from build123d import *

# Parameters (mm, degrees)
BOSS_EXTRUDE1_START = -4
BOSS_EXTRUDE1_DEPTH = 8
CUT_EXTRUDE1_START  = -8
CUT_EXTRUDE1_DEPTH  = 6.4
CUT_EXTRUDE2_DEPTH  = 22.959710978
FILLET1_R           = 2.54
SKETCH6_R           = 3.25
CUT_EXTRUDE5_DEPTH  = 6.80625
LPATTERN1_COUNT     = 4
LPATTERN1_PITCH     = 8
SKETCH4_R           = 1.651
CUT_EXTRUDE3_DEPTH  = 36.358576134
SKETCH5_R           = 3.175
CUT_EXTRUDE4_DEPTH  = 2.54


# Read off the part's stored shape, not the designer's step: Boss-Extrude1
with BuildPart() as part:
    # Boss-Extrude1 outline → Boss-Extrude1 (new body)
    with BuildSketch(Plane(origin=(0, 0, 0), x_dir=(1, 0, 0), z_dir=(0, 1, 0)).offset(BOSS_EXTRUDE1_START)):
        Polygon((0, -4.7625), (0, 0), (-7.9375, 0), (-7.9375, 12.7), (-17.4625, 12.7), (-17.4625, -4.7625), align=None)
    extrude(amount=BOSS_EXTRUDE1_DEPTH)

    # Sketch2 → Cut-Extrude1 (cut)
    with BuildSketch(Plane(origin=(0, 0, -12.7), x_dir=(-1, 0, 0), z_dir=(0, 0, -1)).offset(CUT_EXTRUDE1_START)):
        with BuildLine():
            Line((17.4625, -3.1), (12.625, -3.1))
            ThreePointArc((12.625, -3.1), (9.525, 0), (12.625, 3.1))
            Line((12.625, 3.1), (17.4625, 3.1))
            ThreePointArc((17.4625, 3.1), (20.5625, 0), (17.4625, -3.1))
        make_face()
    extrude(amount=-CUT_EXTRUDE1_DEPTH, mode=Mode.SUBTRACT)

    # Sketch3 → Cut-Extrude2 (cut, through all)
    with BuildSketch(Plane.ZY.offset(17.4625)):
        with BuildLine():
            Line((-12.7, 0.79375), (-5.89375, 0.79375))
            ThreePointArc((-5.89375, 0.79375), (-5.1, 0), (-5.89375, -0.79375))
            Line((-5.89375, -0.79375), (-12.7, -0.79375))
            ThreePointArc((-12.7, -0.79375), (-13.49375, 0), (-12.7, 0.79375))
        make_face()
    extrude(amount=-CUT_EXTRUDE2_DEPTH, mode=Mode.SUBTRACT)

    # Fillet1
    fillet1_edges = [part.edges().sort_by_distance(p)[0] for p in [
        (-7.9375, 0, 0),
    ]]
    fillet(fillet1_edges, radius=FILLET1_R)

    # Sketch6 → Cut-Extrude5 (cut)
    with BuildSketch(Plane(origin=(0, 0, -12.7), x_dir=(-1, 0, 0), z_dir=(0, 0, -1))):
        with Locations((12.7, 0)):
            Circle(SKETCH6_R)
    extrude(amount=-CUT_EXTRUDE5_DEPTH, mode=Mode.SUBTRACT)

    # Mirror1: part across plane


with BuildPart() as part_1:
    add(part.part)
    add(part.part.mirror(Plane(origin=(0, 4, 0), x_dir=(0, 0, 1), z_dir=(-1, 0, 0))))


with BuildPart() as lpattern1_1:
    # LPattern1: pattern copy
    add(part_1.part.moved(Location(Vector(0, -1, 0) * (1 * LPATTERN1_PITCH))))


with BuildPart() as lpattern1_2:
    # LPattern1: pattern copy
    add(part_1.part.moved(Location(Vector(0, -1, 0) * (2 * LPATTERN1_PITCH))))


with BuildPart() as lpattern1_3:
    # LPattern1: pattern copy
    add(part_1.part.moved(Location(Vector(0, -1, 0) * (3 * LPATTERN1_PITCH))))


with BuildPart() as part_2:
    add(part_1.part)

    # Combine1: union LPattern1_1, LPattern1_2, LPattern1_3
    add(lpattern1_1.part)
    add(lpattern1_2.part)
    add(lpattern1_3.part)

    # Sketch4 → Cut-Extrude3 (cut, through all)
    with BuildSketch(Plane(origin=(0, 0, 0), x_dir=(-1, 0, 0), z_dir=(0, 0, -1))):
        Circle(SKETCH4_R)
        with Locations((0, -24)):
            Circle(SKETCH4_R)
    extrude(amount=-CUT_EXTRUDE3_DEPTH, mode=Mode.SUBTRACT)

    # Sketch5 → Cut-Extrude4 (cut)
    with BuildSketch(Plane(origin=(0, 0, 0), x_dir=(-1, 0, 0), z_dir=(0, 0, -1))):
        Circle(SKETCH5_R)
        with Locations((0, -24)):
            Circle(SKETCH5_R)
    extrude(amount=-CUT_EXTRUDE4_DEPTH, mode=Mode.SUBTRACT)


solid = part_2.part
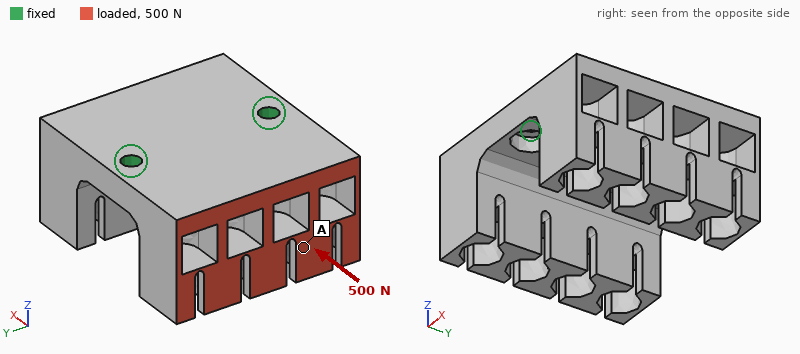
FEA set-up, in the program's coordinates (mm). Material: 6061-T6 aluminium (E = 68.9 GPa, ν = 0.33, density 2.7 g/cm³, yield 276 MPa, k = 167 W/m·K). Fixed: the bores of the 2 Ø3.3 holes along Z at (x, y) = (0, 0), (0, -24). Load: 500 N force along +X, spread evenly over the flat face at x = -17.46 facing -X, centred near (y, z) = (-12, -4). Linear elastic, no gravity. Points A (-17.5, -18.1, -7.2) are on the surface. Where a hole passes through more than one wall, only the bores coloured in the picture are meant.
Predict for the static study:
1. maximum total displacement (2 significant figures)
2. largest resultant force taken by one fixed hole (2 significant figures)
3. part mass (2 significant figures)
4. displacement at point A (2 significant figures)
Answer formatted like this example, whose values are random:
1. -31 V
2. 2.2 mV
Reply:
1. 86 µm
2. 250 N
3. 23 g
4. 72 µm
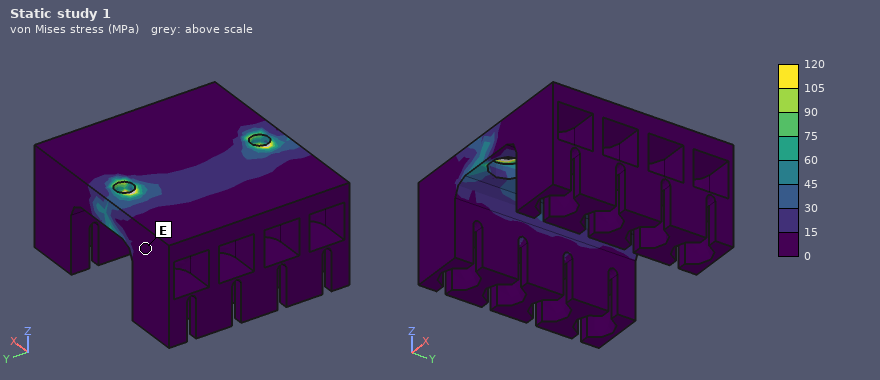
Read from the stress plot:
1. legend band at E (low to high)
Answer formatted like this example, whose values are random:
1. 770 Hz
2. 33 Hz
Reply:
1. 0 to 15 MPa
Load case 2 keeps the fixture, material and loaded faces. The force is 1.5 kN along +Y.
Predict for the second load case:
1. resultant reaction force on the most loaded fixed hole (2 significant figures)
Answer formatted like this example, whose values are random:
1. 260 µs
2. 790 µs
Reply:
1. 1.4 kN
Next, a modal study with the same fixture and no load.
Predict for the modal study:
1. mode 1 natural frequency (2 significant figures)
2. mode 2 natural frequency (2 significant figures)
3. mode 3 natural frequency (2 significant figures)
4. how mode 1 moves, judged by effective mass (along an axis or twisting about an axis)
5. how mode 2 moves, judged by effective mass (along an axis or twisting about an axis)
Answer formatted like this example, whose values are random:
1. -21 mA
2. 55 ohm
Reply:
1. 3200 Hz
2. 6300 Hz
3. 9000 Hz
4. along X
5. along Z
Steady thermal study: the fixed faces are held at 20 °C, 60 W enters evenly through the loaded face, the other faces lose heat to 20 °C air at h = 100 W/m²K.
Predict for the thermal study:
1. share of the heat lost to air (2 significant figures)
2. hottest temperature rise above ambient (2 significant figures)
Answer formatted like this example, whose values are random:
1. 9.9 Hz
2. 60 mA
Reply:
1. 23 %
2. 50 K
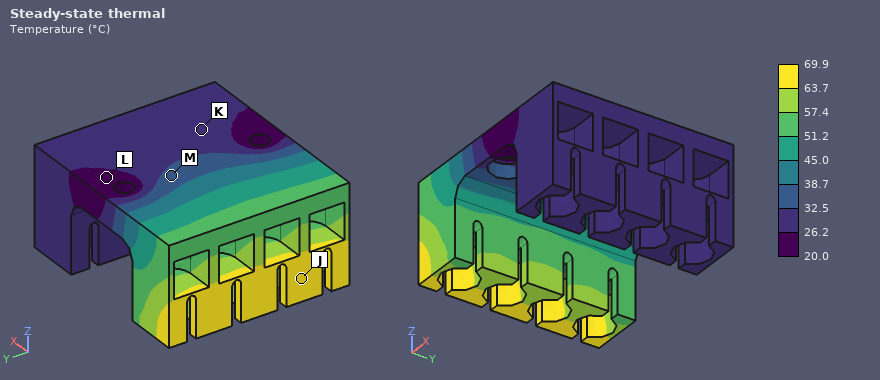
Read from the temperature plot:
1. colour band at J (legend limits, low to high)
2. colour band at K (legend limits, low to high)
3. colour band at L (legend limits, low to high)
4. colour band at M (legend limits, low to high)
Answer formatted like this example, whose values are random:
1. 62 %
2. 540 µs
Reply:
1. 63.7 to 69.9 °C
2. 26.2 to 32.5 °C
3. 20.0 to 26.2 °C
4. 32.5 to 38.7 °C
